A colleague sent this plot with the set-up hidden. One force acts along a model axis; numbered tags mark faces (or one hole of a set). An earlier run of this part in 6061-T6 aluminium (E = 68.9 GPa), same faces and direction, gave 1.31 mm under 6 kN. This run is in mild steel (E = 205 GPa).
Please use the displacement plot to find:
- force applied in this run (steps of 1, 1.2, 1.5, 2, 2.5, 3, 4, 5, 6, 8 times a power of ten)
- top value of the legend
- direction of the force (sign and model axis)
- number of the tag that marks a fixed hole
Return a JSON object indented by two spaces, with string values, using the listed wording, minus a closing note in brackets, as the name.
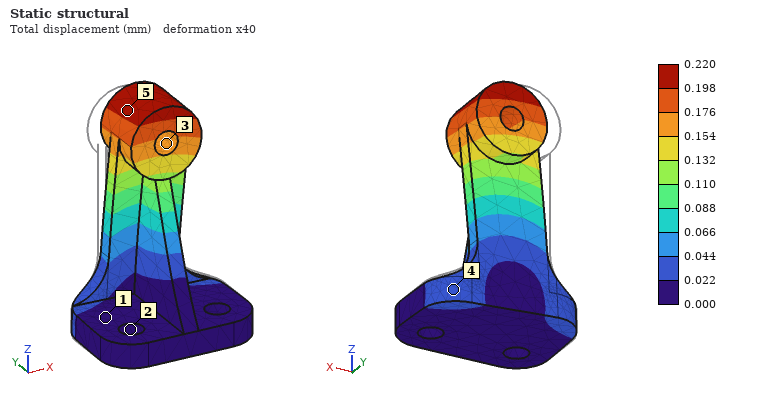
{
  "force applied in this run": "3 kN",
  "top value of the legend": "0.220 mm",
  "direction of the force": "+X",
  "number of the tag that marks a fixed hole": "2"
}
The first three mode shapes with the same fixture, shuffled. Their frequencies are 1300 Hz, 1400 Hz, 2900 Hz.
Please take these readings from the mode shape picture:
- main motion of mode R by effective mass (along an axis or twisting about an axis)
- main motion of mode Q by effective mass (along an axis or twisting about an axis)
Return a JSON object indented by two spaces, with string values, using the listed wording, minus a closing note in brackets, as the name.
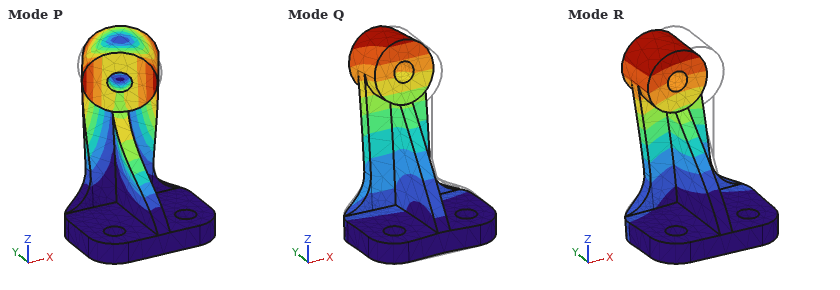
{
  "main motion of mode R by effective mass": "along X",
  "main motion of mode Q by effective mass": "along Y"
}
